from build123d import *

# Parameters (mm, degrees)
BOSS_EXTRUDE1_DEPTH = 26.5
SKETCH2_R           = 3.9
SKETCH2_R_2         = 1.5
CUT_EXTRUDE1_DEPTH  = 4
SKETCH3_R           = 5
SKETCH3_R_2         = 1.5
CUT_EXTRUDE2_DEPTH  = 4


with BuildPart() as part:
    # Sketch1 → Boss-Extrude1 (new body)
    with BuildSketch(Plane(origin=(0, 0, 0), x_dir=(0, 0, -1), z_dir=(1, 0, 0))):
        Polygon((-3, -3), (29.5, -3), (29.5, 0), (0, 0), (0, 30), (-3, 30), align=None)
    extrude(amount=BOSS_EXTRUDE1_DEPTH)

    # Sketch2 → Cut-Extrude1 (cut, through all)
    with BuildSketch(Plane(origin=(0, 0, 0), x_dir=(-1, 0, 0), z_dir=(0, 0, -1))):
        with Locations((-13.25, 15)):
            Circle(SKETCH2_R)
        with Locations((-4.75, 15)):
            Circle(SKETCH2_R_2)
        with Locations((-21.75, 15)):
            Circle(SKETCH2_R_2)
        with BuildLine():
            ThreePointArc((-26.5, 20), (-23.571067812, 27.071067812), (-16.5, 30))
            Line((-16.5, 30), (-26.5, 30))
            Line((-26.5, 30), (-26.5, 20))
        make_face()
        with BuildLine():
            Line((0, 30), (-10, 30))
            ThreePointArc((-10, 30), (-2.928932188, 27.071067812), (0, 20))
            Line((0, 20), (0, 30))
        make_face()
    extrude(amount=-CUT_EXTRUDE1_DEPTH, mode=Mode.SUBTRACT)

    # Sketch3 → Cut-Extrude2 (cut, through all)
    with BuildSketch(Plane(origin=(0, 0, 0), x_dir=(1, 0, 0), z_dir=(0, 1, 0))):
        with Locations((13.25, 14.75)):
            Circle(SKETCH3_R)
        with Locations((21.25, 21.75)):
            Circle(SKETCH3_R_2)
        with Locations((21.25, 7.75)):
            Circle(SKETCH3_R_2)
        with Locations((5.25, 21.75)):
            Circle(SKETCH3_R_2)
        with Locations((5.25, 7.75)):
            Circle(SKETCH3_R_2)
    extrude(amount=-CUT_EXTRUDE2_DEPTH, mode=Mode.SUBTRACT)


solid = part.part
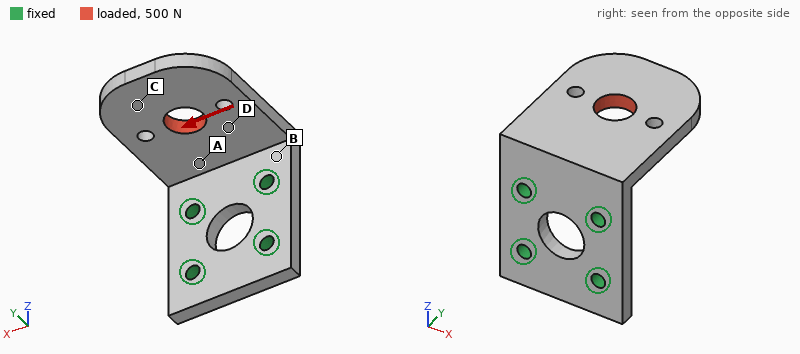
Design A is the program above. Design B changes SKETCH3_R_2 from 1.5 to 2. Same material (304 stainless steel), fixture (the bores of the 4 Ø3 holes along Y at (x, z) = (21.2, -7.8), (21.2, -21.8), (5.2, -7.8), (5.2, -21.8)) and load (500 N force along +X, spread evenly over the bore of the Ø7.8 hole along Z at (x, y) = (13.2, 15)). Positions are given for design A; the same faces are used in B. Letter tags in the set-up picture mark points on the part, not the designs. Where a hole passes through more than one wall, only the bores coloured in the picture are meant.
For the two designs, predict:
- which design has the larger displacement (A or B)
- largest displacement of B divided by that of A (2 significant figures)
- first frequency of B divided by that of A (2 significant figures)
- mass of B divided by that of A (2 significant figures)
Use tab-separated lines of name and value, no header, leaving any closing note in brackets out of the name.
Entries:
which design has the larger displacement	A
largest displacement of B divided by that of A	0.87
first frequency of B divided by that of A	1.0
mass of B divided by that of A	0.98
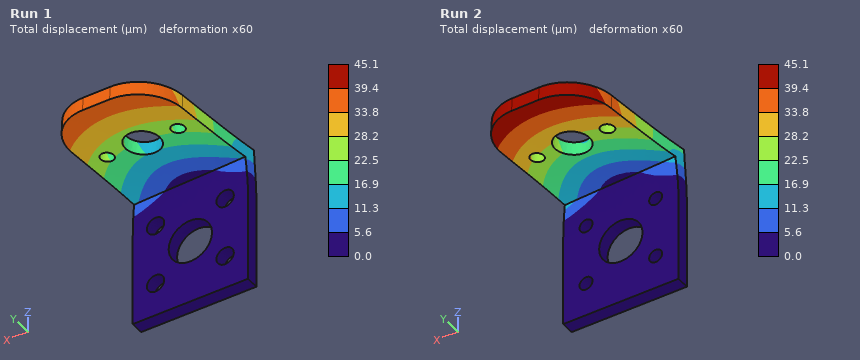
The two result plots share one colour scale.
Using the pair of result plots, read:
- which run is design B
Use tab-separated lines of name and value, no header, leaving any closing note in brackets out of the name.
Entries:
which run is design B	Run 1
